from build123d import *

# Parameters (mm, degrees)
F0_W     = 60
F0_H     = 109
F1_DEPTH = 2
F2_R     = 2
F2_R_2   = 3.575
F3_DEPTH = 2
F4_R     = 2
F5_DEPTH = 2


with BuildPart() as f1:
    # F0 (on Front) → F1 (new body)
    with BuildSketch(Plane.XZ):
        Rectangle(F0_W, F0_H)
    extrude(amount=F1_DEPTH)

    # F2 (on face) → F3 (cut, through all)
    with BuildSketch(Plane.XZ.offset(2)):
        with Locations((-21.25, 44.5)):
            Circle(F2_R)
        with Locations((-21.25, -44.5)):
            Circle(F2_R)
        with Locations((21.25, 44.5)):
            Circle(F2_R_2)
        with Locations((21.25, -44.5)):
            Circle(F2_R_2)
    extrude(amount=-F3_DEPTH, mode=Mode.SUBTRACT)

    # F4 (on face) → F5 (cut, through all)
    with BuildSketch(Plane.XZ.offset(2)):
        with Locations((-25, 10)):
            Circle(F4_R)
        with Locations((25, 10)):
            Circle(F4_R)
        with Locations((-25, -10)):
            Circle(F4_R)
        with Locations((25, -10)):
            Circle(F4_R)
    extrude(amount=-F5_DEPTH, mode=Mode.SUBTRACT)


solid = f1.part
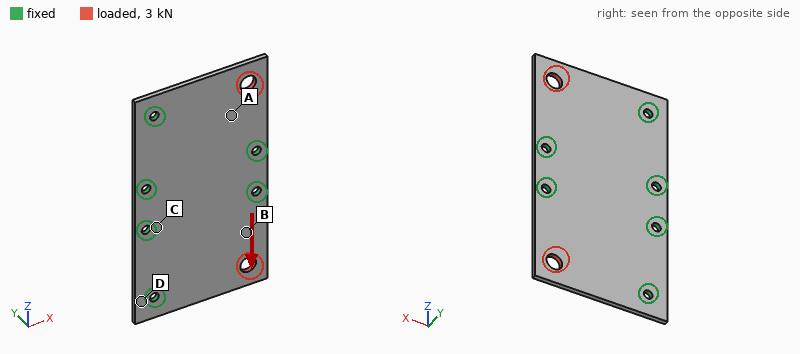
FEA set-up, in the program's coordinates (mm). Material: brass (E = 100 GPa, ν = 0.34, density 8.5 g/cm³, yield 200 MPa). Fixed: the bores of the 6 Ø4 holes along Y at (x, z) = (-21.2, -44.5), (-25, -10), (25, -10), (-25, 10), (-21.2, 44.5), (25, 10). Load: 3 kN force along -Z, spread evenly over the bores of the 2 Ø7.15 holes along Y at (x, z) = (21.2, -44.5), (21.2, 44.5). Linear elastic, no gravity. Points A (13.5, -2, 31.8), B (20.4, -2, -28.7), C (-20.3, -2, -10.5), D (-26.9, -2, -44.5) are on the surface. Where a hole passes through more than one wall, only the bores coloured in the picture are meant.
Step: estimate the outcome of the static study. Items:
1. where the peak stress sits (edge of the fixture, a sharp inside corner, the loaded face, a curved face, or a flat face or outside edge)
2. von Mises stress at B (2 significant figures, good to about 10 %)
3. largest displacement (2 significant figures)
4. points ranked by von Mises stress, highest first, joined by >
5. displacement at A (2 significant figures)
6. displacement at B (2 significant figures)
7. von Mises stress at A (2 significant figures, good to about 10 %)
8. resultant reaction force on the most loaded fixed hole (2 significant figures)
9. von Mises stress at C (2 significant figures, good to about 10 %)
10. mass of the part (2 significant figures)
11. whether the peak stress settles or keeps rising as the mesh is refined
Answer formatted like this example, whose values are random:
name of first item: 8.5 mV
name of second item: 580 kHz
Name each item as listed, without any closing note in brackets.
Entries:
where the peak stress sits: edge of the fixture
von Mises stress at B: 31 MPa
largest displacement: 18 µm
points ranked by von Mises stress, highest first, joined by >: B > A > C > D
displacement at A: 6.7 µm
displacement at B: 7.1 µm
von Mises stress at A: 22 MPa
resultant reaction force on the most loaded fixed hole: 1.1 kN
von Mises stress at C: 11 MPa
mass of the part: 110 g
whether the peak stress settles or keeps rising as the mesh is refined: keeps rising
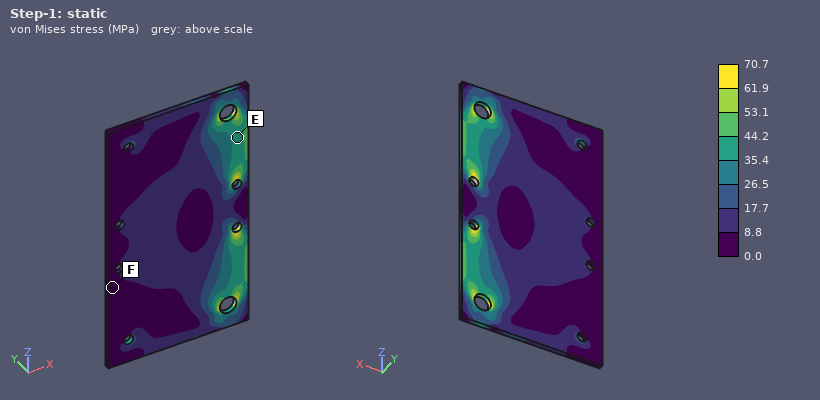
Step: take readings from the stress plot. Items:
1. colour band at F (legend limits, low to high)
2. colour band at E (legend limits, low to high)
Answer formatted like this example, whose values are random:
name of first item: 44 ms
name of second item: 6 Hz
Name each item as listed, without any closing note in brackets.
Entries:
colour band at F: 0.0 to 8.8 MPa
colour band at E: 35.4 to 44.2 MPa
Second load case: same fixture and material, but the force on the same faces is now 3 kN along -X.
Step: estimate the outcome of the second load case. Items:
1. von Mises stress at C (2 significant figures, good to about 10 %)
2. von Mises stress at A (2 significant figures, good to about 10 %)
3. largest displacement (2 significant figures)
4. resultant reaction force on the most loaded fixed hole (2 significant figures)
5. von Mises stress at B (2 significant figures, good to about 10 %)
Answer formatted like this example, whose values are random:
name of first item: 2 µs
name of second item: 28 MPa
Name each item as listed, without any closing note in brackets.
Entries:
von Mises stress at C: 13 MPa
von Mises stress at A: 21 MPa
largest displacement: 18 µm
resultant reaction force on the most loaded fixed hole: 980 N
von Mises stress at B: 11 MPa
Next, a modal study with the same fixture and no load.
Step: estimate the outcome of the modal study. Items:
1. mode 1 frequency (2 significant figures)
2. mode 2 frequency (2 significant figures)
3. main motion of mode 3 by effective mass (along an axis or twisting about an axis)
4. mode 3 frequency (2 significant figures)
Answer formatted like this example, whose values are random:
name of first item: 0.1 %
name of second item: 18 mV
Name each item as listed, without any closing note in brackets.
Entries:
mode 1 frequency: 1000 Hz
mode 2 frequency: 1000 Hz
main motion of mode 3 by effective mass: along Y
mode 3 frequency: 2700 Hz
